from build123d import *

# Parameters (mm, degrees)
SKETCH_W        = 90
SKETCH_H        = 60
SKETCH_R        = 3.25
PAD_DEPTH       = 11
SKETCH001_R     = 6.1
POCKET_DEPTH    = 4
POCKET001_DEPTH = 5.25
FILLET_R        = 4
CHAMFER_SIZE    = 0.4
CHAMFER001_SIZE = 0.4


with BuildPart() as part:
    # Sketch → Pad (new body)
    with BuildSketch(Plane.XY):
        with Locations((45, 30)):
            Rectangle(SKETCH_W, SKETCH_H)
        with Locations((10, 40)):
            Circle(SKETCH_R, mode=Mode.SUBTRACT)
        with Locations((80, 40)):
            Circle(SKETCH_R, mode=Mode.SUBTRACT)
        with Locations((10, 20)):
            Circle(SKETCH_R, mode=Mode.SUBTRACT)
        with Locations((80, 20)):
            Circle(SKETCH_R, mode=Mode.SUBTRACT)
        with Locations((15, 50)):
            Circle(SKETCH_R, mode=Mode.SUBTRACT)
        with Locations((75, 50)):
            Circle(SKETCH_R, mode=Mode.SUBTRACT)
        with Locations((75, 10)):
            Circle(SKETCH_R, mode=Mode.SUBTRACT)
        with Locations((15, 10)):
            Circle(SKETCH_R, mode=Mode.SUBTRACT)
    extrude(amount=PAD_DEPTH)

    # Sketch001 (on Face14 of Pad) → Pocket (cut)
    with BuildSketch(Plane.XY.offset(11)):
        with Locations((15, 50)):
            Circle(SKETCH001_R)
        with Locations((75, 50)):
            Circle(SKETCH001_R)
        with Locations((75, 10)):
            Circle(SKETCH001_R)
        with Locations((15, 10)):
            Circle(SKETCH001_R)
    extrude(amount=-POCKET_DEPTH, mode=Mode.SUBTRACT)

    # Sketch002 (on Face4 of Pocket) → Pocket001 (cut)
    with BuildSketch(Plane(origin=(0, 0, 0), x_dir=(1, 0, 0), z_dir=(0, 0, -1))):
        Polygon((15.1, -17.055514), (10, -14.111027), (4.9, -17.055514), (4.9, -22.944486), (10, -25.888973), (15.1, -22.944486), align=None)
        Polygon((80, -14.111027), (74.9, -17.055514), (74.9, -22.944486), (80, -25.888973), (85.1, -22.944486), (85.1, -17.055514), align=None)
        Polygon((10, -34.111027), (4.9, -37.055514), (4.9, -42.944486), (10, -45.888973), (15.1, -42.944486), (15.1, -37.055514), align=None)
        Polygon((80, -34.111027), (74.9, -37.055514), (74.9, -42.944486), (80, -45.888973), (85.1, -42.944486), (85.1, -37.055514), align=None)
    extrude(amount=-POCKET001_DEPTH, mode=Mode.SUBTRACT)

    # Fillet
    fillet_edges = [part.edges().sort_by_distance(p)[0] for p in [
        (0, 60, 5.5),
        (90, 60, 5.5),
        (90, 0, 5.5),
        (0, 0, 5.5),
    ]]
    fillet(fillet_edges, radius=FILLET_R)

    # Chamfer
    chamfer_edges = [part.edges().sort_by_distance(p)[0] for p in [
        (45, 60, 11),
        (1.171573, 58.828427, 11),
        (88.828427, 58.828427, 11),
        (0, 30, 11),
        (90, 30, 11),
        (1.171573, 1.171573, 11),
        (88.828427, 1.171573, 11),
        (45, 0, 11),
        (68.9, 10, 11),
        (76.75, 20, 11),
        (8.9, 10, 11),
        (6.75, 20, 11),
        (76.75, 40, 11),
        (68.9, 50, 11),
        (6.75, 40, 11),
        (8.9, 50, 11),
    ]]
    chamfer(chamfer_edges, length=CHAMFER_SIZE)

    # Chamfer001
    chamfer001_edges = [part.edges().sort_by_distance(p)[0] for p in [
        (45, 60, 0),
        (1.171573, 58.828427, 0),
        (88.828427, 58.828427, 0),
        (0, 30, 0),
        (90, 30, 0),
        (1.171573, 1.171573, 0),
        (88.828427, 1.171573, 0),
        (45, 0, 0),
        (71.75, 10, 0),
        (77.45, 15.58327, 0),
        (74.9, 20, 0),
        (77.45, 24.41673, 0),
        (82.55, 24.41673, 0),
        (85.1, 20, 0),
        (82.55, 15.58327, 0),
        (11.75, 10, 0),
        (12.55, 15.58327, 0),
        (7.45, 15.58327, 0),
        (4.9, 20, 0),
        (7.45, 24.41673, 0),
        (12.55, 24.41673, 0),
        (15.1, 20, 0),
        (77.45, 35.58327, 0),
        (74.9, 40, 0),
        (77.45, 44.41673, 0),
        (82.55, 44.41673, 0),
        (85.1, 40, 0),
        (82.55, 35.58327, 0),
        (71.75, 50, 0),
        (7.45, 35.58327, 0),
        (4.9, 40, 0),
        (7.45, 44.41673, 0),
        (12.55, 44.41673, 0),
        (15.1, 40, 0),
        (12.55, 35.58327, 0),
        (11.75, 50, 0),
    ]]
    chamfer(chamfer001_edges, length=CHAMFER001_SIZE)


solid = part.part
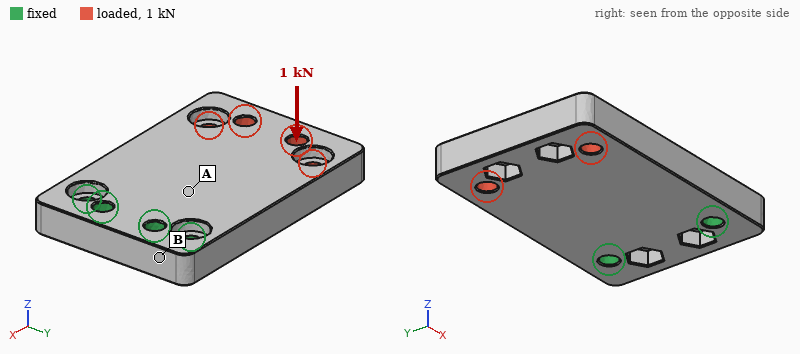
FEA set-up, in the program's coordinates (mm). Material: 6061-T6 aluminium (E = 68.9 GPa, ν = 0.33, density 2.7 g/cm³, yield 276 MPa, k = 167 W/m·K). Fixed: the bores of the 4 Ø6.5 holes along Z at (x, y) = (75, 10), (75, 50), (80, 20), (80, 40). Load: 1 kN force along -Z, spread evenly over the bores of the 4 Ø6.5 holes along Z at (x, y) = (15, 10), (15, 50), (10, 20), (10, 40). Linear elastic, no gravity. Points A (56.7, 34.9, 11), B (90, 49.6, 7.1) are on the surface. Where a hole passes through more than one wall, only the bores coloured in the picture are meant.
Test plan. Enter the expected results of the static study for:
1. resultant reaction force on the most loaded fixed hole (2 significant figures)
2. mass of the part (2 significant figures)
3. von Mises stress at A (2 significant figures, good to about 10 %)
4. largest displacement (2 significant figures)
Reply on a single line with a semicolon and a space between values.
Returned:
2.1 kN; 150 g; 39 MPa; 0.29 mm
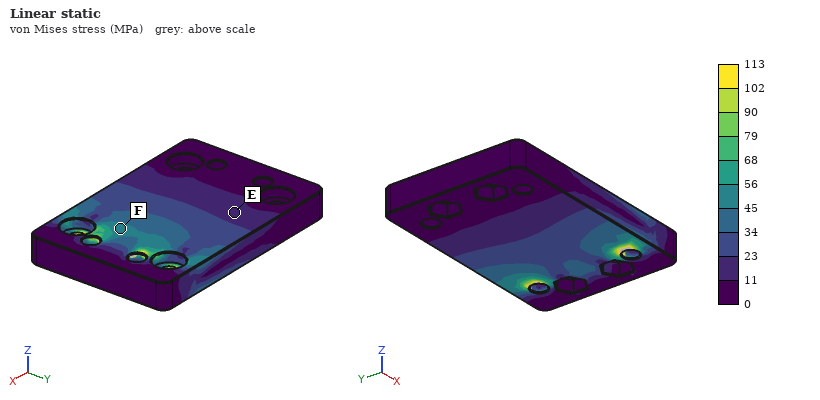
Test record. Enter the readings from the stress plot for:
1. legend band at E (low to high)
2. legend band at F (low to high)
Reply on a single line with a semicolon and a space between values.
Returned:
11 to 23 MPa; 45 to 56 MPa
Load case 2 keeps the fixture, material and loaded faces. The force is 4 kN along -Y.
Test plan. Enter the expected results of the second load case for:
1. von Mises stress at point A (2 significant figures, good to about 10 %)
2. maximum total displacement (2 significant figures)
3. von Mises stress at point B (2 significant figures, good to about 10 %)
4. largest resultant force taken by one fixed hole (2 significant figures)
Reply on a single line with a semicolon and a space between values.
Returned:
14 MPa; 64 µm; 9.2 MPa; 5.4 kN
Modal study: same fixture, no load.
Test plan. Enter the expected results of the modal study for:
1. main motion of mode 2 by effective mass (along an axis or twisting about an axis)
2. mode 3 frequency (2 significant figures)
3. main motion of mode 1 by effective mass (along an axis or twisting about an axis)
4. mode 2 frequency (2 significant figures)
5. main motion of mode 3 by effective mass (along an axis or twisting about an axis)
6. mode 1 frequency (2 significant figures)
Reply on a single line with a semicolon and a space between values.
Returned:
twisting about X; 6000 Hz; along Z; 4100 Hz; along Y; 1500 Hz
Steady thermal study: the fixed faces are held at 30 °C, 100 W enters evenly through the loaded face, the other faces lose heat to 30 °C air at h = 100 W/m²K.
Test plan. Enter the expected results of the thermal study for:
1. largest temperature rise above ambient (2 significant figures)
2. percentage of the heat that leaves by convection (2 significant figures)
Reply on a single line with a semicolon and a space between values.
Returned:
51 K; 32 %
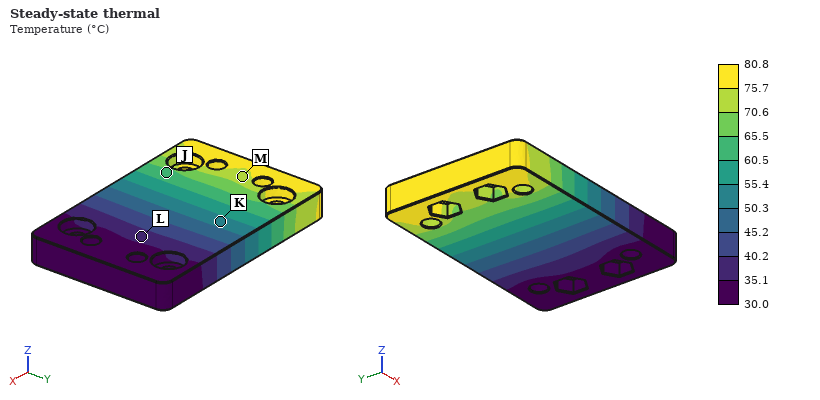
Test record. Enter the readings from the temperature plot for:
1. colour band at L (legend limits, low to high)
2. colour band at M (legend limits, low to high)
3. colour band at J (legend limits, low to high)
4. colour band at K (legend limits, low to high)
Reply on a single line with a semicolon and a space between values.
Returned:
35.1 to 40.2 °C; 70.6 to 75.7 °C; 60.5 to 65.5 °C; 50.3 to 55.4 °C
